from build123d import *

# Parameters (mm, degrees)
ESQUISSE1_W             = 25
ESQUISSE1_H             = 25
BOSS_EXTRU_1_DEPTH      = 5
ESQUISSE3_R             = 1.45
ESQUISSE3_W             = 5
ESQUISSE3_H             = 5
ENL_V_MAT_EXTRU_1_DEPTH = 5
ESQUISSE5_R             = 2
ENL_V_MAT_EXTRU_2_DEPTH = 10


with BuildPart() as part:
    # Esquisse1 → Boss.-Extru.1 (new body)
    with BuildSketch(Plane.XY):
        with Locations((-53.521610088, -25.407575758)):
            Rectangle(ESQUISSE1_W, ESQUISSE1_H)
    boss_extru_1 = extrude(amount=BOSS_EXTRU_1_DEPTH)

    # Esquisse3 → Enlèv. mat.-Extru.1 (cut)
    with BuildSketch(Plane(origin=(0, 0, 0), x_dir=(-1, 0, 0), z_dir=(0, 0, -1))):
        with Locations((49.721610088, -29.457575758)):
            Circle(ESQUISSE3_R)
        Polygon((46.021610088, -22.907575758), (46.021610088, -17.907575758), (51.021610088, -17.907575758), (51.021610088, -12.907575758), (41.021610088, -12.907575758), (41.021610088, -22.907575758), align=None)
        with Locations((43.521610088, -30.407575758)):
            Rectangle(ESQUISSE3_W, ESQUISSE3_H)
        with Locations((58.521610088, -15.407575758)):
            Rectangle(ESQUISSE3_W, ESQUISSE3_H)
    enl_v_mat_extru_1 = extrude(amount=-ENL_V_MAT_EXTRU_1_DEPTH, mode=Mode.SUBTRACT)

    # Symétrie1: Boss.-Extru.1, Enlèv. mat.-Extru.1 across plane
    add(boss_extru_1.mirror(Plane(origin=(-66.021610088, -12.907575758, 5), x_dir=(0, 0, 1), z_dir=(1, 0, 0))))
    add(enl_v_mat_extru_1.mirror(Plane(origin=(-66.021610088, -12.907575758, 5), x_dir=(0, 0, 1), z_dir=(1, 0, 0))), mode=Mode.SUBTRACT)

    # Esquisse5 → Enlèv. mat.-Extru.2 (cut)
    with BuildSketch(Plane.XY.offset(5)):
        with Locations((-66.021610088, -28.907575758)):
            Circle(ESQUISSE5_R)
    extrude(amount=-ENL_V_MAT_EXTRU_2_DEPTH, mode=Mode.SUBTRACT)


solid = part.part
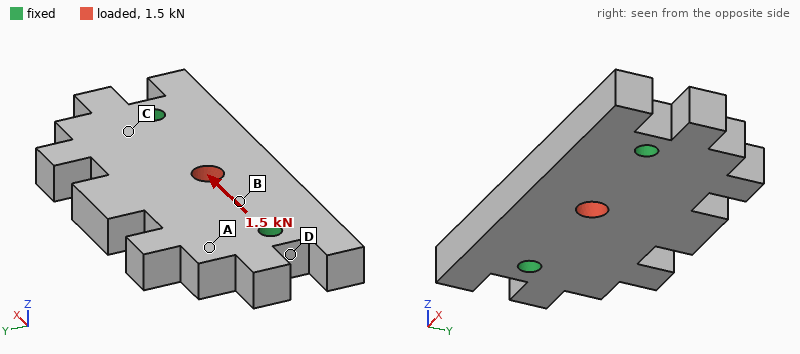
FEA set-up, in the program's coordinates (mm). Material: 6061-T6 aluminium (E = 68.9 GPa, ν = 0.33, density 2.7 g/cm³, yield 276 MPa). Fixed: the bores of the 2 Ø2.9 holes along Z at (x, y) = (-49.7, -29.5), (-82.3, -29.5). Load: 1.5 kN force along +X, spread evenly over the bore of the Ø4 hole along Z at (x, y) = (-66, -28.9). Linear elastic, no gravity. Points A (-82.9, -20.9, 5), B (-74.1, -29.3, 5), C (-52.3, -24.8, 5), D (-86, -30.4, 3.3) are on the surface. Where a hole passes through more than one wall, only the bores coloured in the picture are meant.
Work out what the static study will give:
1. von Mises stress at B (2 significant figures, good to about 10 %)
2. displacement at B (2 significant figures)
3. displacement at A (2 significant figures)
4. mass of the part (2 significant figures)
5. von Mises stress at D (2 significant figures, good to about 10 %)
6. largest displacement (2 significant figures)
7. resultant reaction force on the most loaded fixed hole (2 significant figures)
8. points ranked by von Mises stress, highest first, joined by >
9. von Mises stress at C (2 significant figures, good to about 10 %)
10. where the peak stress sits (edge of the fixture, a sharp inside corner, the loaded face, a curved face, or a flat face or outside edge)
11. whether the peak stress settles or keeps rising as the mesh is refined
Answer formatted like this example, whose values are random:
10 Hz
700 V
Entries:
18 MPa
1.9 µm
1.7 µm
13 g
13 MPa
3.8 µm
750 N
B > D > C > A
6.9 MPa
edge of the fixture
keeps rising
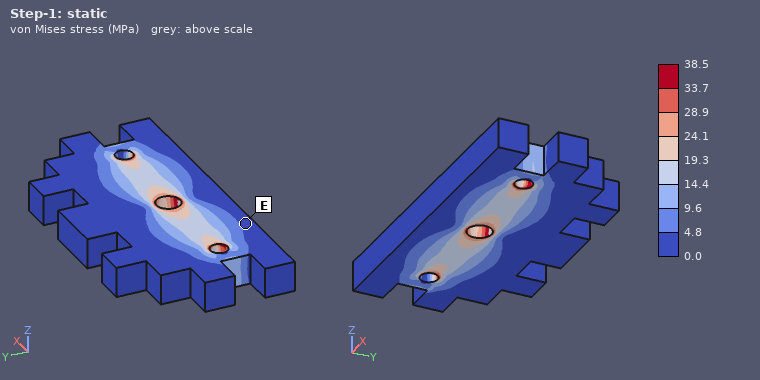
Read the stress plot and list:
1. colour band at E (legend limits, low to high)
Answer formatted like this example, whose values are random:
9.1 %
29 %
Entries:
0.0 to 4.8 MPa
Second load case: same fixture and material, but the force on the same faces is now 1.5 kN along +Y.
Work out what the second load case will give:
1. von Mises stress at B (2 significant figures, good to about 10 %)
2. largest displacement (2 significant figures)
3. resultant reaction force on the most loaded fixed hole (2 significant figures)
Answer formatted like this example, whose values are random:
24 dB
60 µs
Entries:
15 MPa
9.6 µm
760 N
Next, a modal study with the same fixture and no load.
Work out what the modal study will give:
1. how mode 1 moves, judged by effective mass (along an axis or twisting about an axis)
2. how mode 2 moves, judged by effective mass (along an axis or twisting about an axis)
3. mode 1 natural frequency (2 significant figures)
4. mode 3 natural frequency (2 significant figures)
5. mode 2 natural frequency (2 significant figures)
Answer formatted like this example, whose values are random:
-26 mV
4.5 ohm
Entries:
along Z
along Z
11 kHz
22 kHz
19 kHz
